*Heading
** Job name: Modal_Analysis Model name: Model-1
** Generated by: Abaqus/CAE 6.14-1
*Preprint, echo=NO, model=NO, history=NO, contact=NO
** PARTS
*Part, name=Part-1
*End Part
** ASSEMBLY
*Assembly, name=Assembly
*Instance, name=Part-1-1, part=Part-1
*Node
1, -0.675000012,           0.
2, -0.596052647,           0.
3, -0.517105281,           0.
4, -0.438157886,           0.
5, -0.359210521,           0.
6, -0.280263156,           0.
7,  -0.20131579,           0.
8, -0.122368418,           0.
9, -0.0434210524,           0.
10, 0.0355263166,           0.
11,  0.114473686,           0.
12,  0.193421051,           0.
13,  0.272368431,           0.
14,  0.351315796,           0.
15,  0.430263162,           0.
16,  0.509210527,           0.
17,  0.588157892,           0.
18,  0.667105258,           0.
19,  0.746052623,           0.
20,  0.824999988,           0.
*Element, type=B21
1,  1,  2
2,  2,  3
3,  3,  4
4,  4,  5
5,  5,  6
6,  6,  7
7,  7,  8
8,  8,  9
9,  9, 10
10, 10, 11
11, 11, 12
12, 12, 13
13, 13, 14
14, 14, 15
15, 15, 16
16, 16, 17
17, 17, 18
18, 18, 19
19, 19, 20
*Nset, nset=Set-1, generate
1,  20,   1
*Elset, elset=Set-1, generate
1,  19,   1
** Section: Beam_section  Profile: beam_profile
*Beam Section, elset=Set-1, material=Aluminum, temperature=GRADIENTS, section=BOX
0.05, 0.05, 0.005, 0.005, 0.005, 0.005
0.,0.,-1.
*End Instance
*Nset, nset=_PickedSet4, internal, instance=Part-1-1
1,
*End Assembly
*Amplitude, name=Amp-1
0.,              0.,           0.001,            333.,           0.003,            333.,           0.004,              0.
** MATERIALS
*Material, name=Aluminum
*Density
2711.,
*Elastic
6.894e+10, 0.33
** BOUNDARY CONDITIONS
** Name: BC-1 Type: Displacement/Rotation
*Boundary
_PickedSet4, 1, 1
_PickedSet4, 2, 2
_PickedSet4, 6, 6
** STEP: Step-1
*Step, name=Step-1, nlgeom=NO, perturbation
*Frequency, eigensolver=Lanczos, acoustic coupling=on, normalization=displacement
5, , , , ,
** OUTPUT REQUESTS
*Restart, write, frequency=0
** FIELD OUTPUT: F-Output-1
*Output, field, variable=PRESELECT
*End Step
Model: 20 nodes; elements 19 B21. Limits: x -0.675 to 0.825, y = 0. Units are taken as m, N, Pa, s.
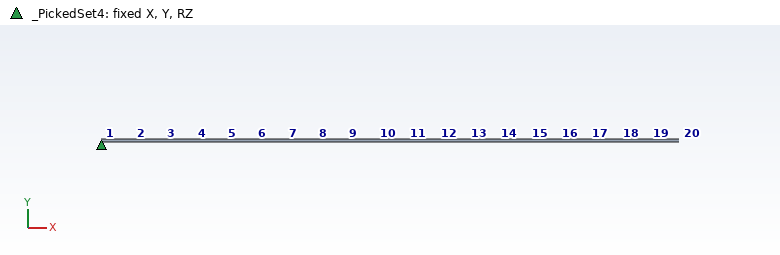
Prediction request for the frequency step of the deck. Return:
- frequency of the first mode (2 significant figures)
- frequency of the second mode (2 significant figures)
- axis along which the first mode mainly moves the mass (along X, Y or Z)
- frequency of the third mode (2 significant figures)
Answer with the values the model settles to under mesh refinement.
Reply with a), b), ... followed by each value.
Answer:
a) 23 Hz
b) 140 Hz
c) along Y
d) 390 Hz
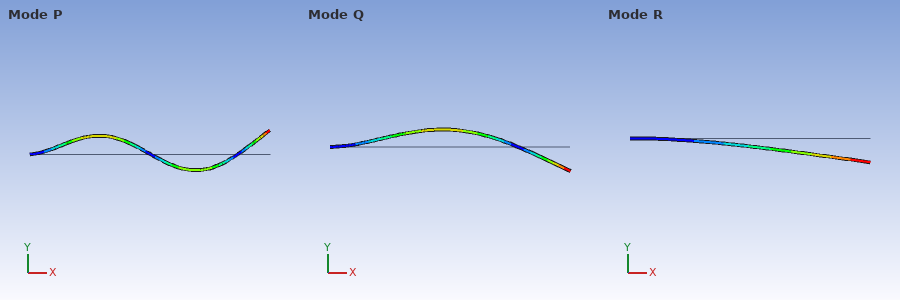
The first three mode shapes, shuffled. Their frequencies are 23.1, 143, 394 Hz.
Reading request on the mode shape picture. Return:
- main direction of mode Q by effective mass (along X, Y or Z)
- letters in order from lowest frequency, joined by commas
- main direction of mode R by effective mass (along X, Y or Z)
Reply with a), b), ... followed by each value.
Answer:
a) along Y
b) R, Q, P
c) along Y
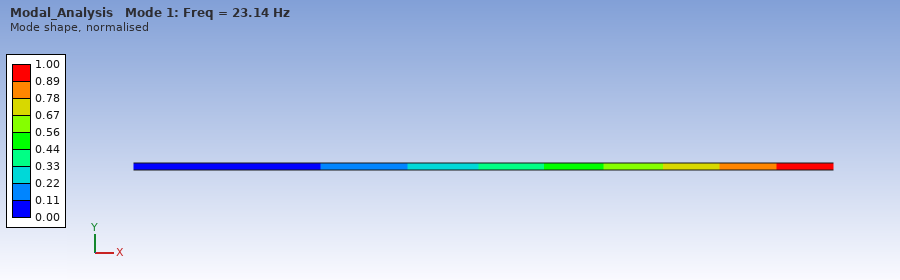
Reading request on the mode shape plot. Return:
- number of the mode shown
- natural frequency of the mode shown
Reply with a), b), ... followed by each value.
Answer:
a) 1
b) 23.14 Hz
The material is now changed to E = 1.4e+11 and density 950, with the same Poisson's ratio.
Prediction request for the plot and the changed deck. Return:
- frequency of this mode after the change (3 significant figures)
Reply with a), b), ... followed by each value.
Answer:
a) 55.7 Hz
